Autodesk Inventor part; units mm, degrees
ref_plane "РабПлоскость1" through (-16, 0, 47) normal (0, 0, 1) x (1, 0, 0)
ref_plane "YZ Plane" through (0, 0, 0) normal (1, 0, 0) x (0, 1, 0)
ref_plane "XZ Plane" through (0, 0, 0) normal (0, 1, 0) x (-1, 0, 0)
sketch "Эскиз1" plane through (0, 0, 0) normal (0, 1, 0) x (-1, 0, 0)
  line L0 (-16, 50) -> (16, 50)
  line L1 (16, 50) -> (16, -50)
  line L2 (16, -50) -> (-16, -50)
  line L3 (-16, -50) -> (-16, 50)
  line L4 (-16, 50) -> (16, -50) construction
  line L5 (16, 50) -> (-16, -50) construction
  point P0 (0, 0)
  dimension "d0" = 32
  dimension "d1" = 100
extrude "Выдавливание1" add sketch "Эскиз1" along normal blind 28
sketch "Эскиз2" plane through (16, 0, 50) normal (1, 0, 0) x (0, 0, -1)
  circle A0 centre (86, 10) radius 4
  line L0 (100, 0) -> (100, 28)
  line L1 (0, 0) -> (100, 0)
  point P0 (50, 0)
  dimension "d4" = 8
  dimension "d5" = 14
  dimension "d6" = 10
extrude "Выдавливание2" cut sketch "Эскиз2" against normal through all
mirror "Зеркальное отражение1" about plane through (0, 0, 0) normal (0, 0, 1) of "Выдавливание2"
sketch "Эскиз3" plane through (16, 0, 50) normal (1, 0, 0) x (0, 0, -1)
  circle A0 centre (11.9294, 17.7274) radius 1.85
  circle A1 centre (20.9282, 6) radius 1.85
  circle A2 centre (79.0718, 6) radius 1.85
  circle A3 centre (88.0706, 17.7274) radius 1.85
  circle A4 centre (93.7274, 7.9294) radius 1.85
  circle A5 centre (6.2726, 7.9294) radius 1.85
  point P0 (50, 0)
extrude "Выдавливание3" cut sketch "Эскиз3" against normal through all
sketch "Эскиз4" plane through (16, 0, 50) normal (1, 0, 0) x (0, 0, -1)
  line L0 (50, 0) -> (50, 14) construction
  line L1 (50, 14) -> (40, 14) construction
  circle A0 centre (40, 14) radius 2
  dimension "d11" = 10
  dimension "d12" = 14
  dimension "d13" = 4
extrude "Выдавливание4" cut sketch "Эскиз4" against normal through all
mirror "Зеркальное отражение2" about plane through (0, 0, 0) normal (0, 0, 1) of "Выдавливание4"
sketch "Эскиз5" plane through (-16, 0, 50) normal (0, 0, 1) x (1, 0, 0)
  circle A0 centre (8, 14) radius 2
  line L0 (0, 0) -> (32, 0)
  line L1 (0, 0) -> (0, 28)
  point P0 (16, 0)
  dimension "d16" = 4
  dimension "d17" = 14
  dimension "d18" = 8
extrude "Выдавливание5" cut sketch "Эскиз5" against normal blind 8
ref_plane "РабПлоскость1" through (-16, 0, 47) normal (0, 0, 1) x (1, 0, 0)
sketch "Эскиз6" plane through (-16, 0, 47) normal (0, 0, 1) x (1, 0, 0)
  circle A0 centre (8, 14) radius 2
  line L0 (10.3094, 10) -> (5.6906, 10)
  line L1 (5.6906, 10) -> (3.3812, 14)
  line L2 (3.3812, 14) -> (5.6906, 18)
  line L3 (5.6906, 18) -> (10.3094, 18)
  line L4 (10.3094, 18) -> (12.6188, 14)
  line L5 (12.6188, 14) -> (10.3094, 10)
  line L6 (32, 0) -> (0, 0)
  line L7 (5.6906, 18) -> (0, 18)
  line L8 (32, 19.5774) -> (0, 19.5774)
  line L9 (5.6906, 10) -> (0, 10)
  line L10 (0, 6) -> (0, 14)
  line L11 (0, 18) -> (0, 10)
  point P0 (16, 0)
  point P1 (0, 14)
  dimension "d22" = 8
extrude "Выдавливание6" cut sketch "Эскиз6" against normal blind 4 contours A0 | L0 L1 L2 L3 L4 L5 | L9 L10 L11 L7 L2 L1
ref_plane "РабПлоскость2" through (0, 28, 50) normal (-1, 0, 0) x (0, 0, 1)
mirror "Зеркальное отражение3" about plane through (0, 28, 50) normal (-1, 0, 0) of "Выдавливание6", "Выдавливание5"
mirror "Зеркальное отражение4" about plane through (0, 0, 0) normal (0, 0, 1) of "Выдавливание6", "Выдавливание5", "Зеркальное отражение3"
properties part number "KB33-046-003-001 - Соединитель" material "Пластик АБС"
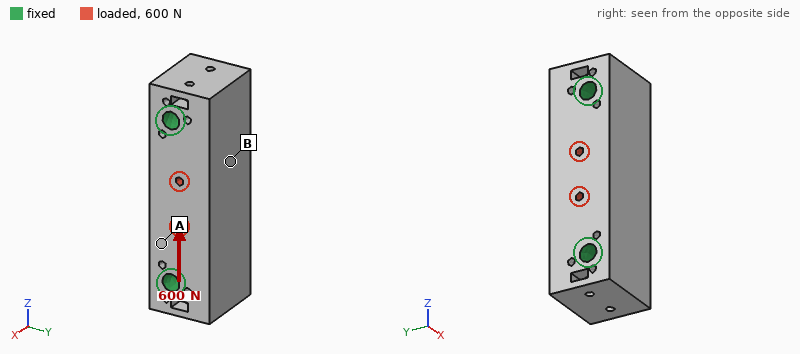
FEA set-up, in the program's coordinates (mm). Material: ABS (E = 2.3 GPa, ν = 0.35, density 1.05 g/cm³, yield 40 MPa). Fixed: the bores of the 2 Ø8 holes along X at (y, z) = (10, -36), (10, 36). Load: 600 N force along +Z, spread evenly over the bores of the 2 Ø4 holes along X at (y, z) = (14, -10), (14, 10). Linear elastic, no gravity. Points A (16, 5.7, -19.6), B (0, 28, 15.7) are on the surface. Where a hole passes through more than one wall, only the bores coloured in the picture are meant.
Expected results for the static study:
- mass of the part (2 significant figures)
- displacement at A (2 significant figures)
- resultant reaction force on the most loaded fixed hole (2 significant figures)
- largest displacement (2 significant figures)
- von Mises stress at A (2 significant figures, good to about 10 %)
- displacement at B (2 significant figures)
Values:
86 g
3.2 µm
300 N
6.9 µm
0.33 MPa
4.0 µm
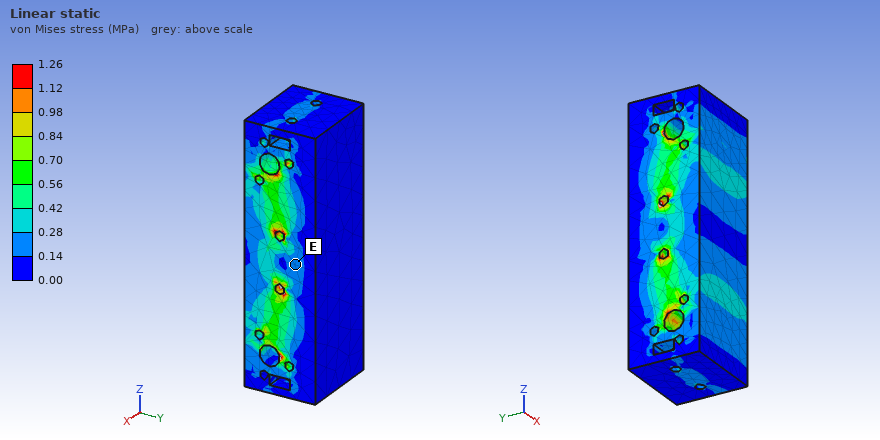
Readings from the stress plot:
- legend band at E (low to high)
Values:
0.14 to 0.28 MPa
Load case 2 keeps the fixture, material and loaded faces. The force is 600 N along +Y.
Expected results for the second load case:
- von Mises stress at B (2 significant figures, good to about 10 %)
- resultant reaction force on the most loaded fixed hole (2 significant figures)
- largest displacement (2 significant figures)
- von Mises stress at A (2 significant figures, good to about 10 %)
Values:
0.85 MPa
320 N
27 µm
0.77 MPa
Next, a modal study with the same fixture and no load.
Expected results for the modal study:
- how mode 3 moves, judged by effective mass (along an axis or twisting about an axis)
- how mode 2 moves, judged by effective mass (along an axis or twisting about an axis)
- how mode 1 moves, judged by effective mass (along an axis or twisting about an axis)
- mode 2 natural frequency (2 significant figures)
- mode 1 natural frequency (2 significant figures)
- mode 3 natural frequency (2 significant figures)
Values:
twisting about Z
along X
along Y
4600 Hz
3900 Hz
5400 Hz
